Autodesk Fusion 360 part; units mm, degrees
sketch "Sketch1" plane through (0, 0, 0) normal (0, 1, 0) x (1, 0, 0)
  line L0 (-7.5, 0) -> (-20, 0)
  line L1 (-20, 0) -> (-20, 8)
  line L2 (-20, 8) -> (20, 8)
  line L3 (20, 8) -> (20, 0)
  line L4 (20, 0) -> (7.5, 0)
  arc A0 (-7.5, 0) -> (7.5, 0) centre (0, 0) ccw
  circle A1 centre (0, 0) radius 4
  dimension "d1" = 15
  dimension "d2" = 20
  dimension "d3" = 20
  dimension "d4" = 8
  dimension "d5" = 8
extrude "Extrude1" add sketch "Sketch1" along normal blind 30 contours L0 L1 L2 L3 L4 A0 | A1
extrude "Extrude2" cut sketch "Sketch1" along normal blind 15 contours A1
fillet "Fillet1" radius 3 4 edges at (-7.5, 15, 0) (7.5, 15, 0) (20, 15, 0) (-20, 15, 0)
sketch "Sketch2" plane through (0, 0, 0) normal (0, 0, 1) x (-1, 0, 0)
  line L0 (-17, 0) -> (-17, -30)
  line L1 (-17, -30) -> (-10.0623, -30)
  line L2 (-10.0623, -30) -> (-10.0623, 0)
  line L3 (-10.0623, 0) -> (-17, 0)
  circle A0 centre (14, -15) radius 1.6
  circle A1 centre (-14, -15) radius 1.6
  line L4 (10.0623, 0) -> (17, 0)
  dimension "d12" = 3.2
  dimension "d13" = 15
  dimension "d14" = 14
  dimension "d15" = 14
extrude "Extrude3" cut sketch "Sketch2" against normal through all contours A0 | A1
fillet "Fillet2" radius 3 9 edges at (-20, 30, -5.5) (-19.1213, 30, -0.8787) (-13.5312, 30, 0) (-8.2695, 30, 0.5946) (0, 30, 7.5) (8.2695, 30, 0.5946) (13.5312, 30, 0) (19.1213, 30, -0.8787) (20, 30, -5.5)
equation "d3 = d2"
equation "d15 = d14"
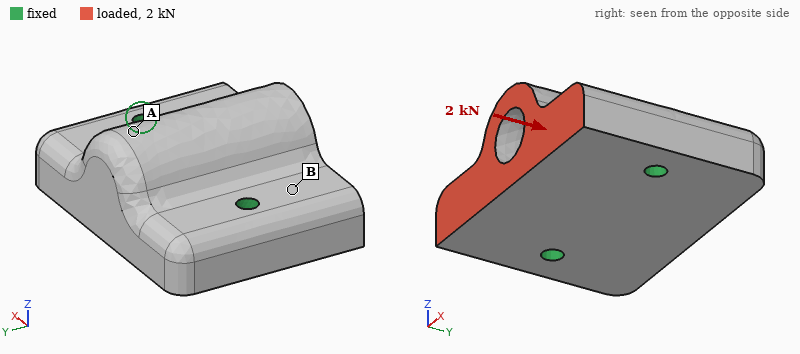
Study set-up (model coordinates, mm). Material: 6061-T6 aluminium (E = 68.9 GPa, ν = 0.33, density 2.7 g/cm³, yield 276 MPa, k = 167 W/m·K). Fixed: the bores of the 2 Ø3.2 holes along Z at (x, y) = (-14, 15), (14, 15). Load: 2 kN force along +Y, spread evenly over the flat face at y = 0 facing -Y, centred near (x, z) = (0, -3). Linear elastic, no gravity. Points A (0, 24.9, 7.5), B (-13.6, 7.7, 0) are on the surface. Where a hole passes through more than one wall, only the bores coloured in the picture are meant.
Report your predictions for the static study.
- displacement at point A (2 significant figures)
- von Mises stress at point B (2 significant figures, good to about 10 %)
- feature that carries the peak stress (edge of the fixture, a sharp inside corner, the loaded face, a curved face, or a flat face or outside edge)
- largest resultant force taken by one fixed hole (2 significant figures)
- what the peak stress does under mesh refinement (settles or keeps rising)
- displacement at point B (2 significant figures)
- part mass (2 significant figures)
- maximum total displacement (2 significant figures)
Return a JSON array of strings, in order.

["3.4 µm", "10 MPa", "edge of the fixture", "1.0 kN", "keeps rising", "1.6 µm", "30 g", "5.2 µm"]
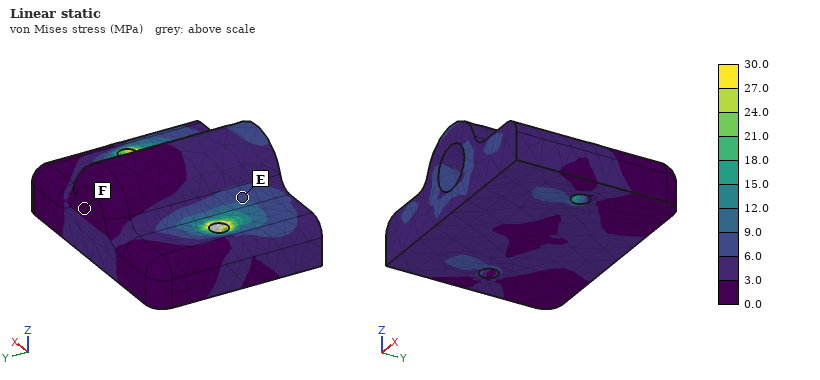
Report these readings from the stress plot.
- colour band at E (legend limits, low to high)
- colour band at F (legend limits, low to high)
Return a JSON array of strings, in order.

["6.0 to 9.0 MPa", "0.0 to 3.0 MPa"]
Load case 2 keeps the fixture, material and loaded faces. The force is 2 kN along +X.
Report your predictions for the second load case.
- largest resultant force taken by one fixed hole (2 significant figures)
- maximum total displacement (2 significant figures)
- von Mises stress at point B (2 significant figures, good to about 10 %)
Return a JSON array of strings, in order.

["1.4 kN", "8.0 µm", "12 MPa"]
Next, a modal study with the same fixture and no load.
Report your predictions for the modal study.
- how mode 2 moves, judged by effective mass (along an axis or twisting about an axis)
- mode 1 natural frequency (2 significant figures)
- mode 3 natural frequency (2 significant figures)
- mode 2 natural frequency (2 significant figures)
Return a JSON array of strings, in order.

["along Z", "14 kHz", "31 kHz", "22 kHz"]
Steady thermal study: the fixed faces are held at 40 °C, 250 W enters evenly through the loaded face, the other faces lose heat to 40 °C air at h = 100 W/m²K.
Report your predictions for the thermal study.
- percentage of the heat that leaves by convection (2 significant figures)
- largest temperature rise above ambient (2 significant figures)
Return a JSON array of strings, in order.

["4.7 %", "82 K"]
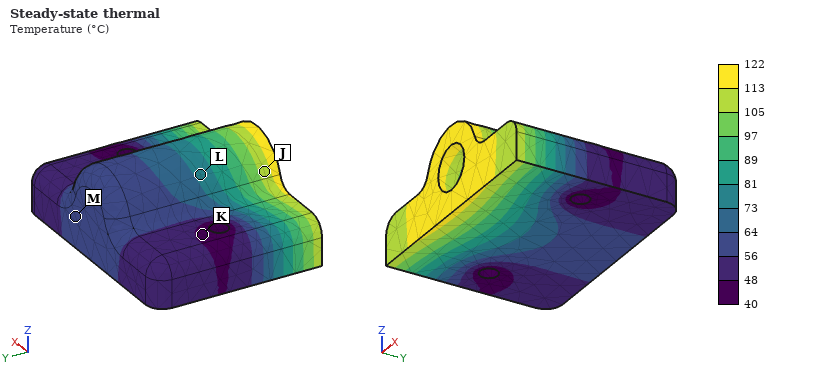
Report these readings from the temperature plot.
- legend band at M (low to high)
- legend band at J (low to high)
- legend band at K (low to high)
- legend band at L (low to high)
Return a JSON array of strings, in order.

["56 to 64 °C", "105 to 113 °C", "40 to 48 °C", "73 to 81 °C"]
